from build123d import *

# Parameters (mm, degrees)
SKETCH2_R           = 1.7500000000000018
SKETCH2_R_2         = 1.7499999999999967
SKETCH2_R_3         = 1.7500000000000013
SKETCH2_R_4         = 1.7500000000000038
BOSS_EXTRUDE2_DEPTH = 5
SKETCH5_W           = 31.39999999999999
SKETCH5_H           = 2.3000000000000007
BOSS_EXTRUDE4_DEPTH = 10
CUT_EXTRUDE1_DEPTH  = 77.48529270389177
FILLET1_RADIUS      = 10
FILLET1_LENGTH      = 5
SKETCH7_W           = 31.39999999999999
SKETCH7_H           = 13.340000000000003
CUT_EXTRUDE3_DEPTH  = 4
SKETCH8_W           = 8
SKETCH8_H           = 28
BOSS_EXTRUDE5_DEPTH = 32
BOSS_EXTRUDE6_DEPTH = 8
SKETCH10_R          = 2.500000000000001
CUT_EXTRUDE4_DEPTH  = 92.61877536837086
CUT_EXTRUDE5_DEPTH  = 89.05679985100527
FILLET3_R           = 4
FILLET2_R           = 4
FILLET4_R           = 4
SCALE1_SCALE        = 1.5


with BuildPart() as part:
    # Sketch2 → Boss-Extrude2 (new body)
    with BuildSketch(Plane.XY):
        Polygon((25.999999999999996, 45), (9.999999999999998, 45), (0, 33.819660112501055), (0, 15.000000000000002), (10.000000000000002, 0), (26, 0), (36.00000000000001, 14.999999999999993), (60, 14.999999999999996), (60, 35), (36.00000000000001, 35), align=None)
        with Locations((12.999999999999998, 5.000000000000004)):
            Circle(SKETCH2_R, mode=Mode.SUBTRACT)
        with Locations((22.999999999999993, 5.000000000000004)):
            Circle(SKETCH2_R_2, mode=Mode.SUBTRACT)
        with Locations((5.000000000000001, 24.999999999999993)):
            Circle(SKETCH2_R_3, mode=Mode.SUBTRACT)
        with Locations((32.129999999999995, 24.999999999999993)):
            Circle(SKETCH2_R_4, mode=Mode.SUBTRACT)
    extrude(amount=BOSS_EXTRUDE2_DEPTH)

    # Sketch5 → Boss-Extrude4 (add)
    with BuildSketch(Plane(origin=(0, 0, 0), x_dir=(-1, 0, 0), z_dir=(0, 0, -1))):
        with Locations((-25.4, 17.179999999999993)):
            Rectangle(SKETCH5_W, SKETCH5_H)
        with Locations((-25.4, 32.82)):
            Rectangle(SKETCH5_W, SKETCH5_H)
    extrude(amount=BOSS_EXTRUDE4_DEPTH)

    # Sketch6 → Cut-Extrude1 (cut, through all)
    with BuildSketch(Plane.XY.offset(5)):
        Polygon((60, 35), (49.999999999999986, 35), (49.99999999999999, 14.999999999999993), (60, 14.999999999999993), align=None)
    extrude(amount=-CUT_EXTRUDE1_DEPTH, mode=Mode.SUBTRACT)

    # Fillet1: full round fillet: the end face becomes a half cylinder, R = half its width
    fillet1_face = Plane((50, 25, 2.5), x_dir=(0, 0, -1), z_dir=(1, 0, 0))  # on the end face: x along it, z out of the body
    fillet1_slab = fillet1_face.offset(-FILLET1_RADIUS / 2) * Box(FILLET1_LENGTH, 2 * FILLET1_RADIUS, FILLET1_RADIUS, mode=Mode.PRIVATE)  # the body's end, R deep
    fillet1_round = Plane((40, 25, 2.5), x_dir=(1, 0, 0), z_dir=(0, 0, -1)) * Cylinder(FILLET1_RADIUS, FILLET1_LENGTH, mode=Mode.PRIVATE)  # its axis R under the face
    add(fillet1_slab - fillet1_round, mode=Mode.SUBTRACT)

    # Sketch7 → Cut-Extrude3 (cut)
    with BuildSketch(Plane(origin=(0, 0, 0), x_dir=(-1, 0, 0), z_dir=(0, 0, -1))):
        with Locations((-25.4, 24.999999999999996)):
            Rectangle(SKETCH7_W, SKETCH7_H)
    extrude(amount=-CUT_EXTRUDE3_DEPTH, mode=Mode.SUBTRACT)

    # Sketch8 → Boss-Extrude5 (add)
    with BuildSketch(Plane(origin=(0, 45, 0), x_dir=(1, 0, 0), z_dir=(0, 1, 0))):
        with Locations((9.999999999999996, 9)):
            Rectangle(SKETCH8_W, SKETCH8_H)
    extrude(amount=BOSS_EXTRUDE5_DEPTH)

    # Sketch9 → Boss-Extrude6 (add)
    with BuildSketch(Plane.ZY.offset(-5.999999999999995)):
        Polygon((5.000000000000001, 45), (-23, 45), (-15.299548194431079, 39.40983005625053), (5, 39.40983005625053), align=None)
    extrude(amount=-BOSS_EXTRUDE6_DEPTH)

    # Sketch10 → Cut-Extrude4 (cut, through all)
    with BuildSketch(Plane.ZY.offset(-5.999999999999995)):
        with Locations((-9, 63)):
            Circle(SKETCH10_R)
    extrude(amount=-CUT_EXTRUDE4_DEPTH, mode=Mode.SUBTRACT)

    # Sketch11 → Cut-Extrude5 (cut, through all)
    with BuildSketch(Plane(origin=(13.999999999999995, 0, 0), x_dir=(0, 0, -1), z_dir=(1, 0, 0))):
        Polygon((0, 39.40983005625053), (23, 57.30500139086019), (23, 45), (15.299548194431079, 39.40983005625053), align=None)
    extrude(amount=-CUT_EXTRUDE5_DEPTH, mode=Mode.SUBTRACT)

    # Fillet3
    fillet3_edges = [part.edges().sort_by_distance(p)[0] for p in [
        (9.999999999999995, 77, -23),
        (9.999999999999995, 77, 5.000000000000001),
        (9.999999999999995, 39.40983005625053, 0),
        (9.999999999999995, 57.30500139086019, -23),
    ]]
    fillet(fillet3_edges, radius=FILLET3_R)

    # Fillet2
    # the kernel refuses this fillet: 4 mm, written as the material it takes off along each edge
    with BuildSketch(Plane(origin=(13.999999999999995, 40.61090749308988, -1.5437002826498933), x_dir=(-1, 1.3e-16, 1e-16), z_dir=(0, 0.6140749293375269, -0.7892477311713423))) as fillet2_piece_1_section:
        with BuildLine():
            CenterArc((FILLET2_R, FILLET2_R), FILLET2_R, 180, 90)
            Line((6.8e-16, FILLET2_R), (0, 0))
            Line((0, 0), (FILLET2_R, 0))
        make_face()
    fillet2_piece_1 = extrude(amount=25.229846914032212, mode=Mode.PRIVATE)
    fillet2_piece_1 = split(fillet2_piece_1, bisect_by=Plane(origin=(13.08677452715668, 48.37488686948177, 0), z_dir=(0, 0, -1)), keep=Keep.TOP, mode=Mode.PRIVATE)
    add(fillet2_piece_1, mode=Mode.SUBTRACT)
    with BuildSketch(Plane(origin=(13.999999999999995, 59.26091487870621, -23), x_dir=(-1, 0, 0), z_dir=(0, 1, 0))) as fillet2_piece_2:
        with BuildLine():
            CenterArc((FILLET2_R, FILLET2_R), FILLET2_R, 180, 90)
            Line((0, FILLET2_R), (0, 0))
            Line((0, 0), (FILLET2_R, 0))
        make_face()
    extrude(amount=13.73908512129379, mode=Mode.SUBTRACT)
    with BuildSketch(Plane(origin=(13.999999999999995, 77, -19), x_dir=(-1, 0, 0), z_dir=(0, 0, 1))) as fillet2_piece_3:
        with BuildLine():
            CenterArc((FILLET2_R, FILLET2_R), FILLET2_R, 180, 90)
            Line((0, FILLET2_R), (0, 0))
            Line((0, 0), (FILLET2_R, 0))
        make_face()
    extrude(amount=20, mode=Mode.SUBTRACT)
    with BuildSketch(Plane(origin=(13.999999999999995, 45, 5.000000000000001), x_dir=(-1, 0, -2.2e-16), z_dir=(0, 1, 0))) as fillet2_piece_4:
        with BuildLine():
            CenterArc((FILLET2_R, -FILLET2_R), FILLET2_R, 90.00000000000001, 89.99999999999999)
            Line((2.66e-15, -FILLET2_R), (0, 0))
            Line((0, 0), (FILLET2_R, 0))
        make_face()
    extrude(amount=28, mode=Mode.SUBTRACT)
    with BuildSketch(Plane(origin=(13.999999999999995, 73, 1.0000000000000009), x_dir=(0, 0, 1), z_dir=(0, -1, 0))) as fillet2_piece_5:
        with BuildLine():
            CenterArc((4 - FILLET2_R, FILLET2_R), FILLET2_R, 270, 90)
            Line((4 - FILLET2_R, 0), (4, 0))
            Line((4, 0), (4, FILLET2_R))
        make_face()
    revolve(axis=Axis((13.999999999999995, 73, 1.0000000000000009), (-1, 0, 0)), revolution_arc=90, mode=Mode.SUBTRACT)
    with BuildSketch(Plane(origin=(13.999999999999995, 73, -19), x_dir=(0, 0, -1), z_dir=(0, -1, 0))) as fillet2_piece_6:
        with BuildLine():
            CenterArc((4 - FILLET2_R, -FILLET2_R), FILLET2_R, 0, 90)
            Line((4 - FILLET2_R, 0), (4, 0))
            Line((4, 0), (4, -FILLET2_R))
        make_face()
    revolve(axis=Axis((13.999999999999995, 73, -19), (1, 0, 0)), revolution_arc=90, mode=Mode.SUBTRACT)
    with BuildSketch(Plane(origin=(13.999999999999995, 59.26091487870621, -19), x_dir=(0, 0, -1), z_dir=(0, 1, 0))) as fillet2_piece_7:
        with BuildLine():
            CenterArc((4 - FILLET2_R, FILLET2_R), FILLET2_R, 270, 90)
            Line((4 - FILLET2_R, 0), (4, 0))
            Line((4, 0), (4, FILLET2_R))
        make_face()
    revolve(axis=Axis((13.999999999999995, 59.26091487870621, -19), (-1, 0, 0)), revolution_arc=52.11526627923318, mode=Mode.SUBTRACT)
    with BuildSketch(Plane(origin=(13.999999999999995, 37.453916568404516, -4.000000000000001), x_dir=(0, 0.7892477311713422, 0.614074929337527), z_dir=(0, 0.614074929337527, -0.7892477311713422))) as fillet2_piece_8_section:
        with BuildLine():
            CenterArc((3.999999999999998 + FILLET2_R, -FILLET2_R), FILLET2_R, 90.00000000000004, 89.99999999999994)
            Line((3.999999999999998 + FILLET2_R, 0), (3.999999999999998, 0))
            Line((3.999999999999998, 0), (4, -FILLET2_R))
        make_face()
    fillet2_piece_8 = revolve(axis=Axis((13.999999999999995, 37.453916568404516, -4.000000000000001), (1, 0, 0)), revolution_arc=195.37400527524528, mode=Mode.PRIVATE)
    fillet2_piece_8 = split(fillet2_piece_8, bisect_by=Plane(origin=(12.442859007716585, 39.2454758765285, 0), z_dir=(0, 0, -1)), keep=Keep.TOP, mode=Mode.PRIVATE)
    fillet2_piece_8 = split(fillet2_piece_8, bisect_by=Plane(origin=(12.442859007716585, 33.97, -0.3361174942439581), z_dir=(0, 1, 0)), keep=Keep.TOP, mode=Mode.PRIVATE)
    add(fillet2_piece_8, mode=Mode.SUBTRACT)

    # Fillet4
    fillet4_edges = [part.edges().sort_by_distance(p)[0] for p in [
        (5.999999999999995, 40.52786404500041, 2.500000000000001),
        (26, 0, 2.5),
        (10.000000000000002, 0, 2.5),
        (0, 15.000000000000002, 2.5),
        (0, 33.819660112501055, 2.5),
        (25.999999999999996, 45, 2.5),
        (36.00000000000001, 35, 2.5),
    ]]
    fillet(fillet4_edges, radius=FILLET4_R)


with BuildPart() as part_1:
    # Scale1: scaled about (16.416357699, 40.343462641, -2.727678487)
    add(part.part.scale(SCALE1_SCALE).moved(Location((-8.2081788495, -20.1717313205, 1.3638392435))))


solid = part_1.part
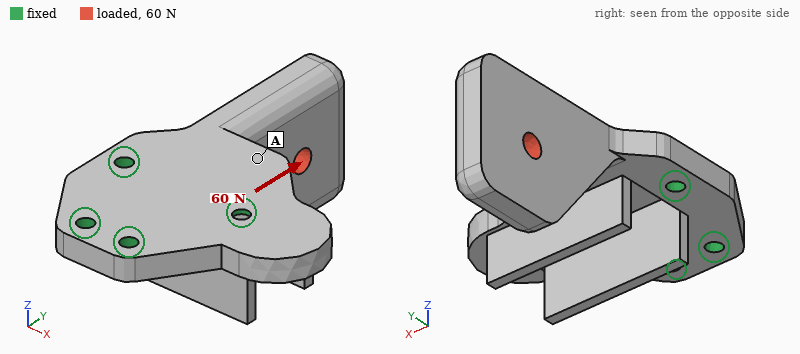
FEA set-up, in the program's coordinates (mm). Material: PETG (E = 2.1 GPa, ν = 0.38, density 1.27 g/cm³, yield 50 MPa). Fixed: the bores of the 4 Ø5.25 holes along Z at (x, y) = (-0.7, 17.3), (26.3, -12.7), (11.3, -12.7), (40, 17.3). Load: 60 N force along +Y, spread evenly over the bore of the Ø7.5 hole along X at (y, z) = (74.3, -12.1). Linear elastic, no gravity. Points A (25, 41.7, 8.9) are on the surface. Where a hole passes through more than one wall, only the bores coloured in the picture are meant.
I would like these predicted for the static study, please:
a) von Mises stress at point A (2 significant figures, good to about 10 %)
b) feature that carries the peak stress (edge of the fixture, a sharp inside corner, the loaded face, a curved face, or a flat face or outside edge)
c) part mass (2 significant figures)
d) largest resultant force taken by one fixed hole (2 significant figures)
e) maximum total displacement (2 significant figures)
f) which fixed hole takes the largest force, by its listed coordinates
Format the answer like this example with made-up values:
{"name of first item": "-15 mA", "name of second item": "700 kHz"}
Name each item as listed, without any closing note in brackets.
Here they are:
{"von Mises stress at point A": "1.1 MPa", "feature that carries the peak stress": "a flat face or outside edge", "part mass": "59 g", "largest resultant force taken by one fixed hole": "67 N", "maximum total displacement": "1.5 mm", "which fixed hole takes the largest force, by its listed coordinates": "(-0.7, 17.3)"}
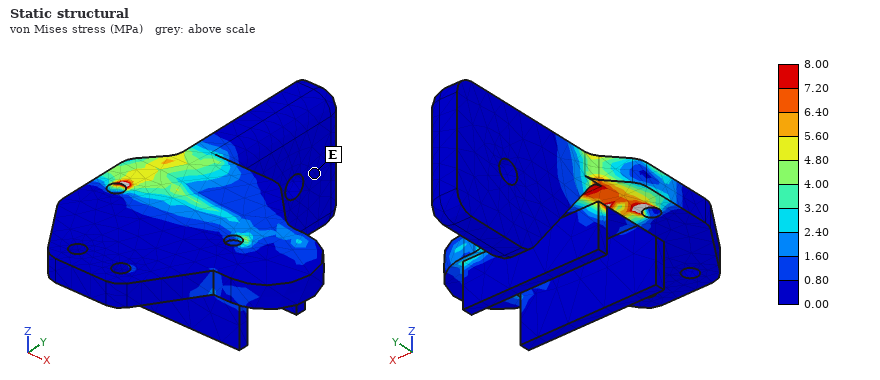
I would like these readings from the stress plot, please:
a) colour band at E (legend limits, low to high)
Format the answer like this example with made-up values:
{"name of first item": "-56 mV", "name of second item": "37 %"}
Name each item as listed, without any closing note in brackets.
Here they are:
{"colour band at E": "0.00 to 0.80 MPa"}
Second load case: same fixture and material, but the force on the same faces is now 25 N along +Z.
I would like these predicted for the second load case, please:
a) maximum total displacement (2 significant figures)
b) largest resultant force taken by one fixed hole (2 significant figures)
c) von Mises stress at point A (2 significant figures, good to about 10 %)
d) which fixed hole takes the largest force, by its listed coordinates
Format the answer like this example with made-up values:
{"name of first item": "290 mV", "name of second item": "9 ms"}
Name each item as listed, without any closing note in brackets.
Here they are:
{"maximum total displacement": "1.5 mm", "largest resultant force taken by one fixed hole": "41 N", "von Mises stress at point A": "1.1 MPa", "which fixed hole takes the largest force, by its listed coordinates": "(-0.7, 17.3)"}
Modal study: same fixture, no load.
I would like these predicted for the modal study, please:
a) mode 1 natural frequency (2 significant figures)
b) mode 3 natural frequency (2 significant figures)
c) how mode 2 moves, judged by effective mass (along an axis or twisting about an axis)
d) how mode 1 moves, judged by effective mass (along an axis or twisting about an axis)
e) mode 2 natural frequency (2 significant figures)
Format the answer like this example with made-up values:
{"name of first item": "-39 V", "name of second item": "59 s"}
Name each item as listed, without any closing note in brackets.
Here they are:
{"mode 1 natural frequency": "150 Hz", "mode 3 natural frequency": "730 Hz", "how mode 2 moves, judged by effective mass": "along X", "how mode 1 moves, judged by effective mass": "along Z", "mode 2 natural frequency": "350 Hz"}
